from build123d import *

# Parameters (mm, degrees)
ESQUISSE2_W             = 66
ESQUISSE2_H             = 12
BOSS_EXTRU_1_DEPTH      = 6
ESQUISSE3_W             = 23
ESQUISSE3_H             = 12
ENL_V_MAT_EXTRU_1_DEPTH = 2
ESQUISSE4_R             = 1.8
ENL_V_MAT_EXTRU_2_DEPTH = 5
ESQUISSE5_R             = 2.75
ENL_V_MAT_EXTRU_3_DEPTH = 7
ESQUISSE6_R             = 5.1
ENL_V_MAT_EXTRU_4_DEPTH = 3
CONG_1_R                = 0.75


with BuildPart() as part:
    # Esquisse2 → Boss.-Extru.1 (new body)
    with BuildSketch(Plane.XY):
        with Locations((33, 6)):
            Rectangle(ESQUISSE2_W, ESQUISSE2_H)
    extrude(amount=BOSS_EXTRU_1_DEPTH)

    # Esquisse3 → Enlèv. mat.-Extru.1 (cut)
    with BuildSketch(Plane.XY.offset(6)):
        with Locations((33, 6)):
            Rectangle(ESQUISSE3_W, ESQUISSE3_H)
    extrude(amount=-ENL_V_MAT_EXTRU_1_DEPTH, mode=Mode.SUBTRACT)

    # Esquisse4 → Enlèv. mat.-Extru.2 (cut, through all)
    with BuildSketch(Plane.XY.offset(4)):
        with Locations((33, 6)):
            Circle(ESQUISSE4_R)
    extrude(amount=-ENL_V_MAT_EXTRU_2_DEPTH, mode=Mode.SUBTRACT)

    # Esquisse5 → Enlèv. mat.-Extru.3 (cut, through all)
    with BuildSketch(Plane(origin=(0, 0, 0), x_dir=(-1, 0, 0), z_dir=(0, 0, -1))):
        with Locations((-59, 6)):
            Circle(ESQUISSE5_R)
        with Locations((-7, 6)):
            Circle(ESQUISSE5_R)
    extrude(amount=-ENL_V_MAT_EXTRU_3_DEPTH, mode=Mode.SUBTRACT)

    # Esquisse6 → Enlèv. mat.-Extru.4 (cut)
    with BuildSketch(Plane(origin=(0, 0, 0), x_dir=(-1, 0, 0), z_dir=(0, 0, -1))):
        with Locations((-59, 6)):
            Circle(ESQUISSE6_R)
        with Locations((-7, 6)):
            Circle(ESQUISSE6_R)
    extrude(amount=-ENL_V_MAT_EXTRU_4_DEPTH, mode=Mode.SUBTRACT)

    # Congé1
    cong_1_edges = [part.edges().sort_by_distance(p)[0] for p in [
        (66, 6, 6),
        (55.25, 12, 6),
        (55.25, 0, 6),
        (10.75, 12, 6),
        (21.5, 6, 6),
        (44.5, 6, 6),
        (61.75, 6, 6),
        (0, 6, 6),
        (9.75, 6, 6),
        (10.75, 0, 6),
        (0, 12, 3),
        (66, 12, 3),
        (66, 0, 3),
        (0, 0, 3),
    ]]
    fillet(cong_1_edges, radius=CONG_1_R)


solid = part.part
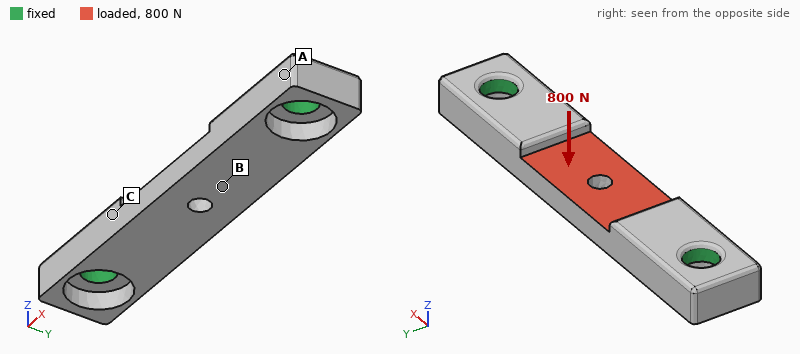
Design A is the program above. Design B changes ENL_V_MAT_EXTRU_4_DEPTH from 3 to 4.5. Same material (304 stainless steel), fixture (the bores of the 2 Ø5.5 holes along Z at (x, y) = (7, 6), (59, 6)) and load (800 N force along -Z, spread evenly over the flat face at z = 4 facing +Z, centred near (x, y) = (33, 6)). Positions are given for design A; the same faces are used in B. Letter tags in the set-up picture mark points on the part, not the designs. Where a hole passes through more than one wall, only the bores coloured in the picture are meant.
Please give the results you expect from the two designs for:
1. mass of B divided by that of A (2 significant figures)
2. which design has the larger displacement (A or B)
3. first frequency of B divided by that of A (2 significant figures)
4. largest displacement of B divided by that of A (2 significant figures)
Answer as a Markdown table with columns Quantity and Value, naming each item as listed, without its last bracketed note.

| Quantity | Value |
|---|---|
| mass of B divided by that of A | 0.95 |
| which design has the larger displacement | B |
| first frequency of B divided by that of A | 0.84 |
| largest displacement of B divided by that of A | 1.3 |
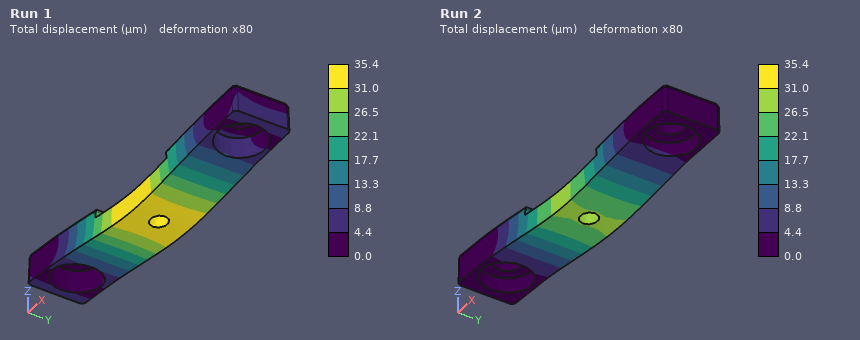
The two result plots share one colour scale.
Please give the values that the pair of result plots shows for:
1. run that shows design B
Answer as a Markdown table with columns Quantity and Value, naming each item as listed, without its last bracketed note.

| Quantity | Value |
|---|---|
| run that shows design B | Run 1 |
